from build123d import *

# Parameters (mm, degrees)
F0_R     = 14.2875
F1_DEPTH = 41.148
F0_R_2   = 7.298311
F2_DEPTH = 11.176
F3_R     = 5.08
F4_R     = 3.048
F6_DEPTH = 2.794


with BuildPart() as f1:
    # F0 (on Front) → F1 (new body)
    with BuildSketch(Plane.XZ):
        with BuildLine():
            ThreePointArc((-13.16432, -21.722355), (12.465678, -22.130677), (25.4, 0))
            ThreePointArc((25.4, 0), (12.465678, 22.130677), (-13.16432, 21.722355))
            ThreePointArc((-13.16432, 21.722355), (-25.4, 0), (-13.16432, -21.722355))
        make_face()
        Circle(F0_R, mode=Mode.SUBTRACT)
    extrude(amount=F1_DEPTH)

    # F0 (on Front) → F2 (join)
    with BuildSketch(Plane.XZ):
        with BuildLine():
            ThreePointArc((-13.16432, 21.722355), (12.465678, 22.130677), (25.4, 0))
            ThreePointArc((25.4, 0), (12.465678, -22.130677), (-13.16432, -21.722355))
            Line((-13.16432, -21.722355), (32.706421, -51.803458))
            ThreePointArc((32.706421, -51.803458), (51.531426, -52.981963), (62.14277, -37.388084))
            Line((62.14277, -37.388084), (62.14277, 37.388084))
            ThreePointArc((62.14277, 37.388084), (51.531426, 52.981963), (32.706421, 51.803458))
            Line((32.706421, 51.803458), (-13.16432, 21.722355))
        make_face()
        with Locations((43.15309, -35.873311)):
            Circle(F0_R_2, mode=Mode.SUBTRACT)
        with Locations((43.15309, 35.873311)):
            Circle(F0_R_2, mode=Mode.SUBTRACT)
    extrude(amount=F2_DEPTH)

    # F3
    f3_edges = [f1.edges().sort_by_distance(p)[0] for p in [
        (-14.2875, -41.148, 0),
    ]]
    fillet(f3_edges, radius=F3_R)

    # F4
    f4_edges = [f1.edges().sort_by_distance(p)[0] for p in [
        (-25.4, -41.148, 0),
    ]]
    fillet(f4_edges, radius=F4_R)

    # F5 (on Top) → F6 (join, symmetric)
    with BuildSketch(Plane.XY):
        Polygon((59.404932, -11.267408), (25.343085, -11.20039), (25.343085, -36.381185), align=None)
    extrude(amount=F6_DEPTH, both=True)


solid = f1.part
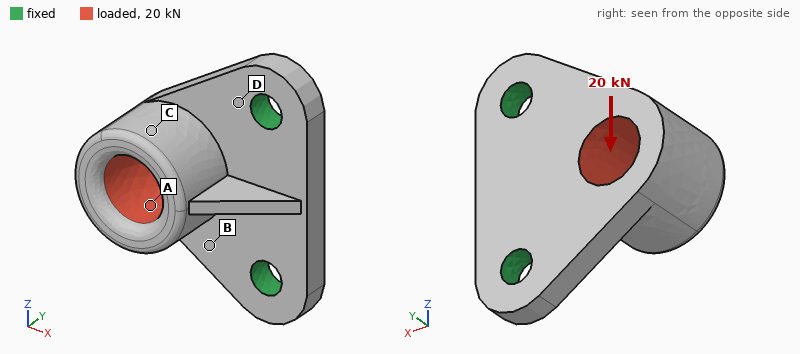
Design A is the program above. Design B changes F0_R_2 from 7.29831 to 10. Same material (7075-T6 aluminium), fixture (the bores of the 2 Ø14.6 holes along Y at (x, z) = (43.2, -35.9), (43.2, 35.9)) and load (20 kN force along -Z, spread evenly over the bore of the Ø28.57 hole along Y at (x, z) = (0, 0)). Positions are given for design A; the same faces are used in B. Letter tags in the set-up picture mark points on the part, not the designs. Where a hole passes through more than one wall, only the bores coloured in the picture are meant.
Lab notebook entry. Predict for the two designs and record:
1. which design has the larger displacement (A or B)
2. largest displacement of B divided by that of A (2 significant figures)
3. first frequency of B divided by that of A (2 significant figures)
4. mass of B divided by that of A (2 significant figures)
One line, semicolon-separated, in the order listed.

A; 0.87; 1.1; 0.97
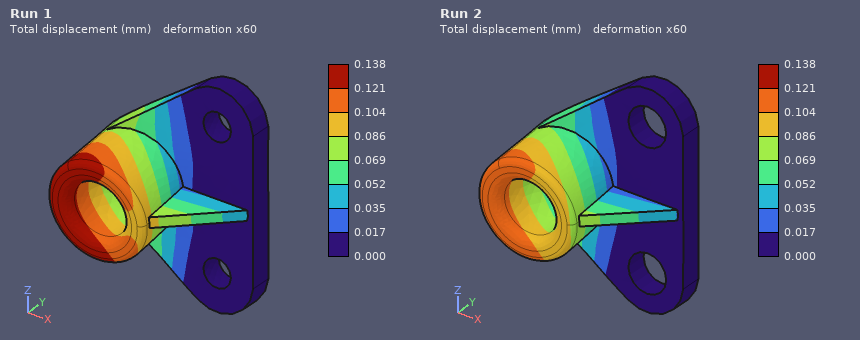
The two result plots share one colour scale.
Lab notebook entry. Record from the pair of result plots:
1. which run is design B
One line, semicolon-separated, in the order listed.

Run 2
